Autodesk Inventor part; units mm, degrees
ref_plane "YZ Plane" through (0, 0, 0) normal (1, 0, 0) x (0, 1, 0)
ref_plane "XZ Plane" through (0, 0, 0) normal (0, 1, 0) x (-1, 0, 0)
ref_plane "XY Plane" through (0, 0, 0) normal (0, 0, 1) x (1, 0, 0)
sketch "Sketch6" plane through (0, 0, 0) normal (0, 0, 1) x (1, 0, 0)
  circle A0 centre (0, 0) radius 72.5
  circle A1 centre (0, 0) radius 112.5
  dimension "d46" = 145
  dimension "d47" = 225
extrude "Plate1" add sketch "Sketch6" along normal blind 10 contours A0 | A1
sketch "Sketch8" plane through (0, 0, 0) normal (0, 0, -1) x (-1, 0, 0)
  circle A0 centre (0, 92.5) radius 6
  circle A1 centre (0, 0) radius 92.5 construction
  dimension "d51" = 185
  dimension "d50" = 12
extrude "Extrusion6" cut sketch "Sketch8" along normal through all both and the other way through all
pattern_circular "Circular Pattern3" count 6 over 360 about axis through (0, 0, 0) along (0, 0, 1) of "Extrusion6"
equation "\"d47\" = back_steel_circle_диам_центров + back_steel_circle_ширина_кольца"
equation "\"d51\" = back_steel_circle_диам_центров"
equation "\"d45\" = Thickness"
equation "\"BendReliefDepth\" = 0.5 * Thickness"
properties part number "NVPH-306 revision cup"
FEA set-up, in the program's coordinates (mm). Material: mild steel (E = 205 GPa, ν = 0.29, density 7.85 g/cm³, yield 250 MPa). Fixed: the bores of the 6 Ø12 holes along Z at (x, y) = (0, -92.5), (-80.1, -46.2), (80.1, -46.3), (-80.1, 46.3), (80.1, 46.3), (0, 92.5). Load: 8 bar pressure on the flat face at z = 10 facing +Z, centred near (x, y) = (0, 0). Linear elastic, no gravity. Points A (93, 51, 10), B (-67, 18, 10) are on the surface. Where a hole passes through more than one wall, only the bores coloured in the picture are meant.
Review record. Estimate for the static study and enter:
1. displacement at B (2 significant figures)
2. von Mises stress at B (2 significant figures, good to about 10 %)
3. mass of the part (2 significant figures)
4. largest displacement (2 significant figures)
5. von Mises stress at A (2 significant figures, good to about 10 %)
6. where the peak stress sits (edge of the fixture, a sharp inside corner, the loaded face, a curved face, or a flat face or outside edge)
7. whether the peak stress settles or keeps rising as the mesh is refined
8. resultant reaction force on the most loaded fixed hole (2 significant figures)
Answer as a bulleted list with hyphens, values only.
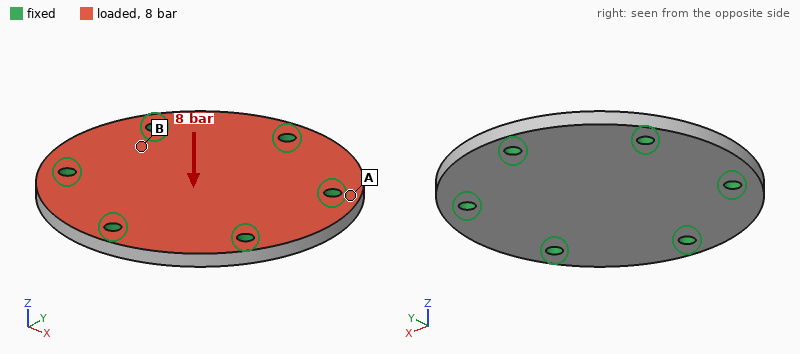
- 18 µm
- 24 MPa
- 3.1 kg
- 60 µm
- 10 MPa
- edge of the fixture
- keeps rising
- 5.2 kN
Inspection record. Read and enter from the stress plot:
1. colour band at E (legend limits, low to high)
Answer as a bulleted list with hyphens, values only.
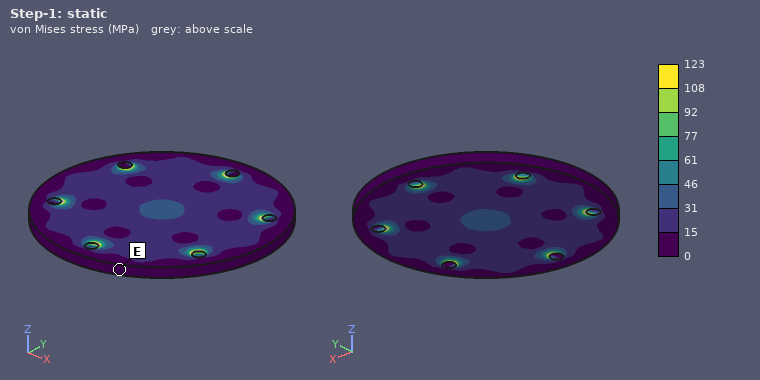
- 0 to 15 MPa
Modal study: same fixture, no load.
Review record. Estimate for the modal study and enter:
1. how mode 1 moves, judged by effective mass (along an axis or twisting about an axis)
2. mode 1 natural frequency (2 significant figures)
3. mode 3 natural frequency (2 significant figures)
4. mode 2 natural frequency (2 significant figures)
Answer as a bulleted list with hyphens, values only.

- along Z
- 2500 Hz
- 5000 Hz
- 5000 Hz
